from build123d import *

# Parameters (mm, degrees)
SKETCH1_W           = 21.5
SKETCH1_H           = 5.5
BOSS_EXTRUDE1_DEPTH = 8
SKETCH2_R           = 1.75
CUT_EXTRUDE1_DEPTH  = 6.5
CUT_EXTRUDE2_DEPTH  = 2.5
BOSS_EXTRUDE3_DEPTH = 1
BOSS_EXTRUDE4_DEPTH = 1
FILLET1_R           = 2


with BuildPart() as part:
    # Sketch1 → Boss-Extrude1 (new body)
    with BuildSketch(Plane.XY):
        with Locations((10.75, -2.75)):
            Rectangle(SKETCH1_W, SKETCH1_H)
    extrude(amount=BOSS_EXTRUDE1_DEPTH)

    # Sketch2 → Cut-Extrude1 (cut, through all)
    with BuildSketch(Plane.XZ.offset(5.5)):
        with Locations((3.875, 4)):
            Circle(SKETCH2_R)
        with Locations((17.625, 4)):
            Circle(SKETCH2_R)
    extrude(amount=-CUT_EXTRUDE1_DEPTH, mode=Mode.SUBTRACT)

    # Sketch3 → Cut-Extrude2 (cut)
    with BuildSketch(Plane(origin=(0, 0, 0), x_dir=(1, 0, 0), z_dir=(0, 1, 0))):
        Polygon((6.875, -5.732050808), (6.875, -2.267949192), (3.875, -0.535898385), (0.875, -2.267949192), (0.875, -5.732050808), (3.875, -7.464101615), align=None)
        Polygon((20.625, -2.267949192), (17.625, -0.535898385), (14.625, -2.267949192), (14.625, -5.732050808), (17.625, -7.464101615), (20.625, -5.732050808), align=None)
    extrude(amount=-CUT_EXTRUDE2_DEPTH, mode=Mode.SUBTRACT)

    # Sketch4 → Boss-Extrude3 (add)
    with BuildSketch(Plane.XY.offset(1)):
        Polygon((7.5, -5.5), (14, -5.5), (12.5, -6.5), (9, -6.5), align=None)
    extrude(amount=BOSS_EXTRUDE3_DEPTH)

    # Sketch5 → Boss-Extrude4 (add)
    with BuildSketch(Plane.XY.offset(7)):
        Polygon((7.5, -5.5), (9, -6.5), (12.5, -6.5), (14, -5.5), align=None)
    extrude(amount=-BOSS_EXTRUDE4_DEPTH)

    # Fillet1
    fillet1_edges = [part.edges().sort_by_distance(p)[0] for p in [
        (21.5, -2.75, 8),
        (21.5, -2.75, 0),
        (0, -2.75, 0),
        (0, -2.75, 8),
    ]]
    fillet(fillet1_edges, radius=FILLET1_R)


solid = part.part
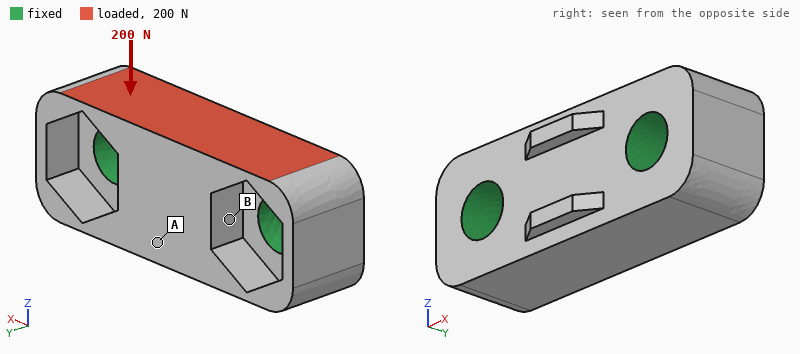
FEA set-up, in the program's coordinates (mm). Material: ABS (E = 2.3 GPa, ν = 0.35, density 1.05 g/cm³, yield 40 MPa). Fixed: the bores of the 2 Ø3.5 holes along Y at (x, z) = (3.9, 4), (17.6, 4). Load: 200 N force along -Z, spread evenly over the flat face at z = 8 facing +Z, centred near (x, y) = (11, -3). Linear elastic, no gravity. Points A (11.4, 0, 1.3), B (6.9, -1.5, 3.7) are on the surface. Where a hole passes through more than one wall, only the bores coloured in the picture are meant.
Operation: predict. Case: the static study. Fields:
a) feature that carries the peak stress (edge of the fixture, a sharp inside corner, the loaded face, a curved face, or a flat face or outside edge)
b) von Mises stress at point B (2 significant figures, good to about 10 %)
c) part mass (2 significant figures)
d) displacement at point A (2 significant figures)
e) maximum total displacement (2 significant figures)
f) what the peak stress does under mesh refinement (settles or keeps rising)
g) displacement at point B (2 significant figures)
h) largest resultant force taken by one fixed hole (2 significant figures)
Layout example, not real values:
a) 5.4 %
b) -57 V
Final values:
a) edge of the fixture
b) 4.1 MPa
c) 0.76 g
d) 26 µm
e) 42 µm
f) keeps rising
g) 18 µm
h) 100 N
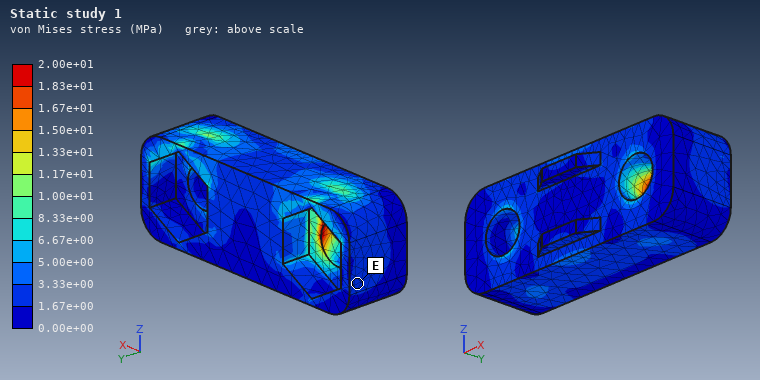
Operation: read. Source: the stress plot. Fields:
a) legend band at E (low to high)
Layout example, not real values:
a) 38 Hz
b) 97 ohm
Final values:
a) 1.67e+00 to 3.33e+00 MPa
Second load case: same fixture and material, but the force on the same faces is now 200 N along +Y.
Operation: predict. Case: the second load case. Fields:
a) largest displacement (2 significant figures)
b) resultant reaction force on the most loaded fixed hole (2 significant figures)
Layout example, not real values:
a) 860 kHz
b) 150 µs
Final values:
a) 73 µm
b) 100 N
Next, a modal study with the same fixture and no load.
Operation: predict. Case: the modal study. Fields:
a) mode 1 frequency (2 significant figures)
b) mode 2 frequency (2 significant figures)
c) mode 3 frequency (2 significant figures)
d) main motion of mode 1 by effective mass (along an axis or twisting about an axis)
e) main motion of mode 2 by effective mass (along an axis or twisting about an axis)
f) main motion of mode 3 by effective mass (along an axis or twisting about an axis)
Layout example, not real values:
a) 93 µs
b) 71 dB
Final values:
a) 18 kHz
b) 23 kHz
c) 27 kHz
d) along Z
e) along Y
f) along Z
